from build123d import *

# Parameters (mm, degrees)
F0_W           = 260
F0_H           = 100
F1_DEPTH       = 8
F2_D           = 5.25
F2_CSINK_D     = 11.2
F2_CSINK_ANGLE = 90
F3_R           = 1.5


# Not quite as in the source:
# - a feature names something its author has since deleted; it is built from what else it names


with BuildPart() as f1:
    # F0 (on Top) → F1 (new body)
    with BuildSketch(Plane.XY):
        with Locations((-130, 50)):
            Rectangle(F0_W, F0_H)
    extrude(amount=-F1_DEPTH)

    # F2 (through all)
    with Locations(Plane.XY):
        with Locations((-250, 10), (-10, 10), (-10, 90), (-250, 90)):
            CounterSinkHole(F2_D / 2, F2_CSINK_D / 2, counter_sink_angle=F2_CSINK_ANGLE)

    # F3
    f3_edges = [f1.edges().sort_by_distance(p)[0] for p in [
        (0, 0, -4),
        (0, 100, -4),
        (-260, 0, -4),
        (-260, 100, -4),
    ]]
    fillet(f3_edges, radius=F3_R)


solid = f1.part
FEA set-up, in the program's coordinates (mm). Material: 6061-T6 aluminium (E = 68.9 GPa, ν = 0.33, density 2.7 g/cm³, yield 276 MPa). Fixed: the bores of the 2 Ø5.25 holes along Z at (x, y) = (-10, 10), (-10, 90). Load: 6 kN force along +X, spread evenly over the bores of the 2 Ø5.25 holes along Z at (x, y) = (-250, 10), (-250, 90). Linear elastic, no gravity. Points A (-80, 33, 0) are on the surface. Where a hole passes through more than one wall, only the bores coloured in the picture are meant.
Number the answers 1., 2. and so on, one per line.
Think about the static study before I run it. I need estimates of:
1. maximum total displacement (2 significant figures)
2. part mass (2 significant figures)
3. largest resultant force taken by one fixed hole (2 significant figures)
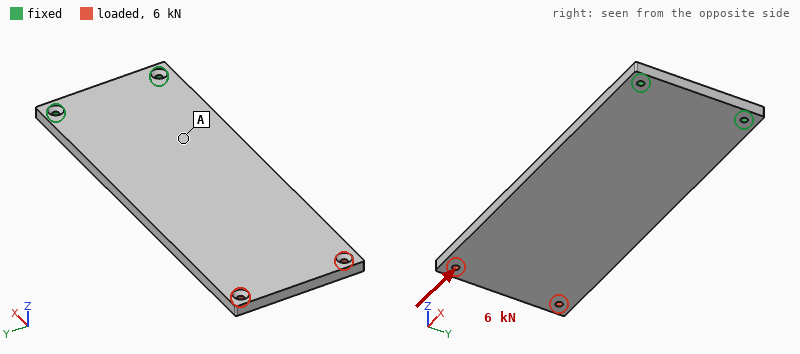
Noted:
1. 0.99 mm
2. 560 g
3. 3.1 kN
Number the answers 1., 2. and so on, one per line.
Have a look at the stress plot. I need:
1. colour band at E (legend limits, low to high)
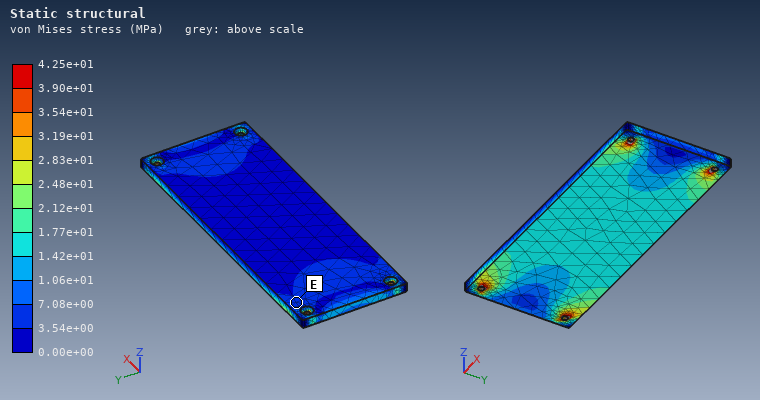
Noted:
1. 3.54e+00 to 7.08e+00 MPa
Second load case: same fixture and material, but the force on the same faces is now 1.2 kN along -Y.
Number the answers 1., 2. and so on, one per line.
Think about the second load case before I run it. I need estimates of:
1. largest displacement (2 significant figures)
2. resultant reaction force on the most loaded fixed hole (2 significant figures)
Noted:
1. 0.18 mm
2. 3.6 kN
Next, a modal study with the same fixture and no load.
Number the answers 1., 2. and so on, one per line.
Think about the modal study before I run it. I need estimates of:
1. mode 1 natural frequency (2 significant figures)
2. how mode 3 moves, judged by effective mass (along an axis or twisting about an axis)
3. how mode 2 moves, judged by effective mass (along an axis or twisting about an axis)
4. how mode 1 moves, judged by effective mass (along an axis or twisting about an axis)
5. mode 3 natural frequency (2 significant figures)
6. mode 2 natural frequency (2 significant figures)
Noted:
1. 91 Hz
2. along Z
3. twisting about X
4. along Z
5. 590 Hz
6. 530 Hz
